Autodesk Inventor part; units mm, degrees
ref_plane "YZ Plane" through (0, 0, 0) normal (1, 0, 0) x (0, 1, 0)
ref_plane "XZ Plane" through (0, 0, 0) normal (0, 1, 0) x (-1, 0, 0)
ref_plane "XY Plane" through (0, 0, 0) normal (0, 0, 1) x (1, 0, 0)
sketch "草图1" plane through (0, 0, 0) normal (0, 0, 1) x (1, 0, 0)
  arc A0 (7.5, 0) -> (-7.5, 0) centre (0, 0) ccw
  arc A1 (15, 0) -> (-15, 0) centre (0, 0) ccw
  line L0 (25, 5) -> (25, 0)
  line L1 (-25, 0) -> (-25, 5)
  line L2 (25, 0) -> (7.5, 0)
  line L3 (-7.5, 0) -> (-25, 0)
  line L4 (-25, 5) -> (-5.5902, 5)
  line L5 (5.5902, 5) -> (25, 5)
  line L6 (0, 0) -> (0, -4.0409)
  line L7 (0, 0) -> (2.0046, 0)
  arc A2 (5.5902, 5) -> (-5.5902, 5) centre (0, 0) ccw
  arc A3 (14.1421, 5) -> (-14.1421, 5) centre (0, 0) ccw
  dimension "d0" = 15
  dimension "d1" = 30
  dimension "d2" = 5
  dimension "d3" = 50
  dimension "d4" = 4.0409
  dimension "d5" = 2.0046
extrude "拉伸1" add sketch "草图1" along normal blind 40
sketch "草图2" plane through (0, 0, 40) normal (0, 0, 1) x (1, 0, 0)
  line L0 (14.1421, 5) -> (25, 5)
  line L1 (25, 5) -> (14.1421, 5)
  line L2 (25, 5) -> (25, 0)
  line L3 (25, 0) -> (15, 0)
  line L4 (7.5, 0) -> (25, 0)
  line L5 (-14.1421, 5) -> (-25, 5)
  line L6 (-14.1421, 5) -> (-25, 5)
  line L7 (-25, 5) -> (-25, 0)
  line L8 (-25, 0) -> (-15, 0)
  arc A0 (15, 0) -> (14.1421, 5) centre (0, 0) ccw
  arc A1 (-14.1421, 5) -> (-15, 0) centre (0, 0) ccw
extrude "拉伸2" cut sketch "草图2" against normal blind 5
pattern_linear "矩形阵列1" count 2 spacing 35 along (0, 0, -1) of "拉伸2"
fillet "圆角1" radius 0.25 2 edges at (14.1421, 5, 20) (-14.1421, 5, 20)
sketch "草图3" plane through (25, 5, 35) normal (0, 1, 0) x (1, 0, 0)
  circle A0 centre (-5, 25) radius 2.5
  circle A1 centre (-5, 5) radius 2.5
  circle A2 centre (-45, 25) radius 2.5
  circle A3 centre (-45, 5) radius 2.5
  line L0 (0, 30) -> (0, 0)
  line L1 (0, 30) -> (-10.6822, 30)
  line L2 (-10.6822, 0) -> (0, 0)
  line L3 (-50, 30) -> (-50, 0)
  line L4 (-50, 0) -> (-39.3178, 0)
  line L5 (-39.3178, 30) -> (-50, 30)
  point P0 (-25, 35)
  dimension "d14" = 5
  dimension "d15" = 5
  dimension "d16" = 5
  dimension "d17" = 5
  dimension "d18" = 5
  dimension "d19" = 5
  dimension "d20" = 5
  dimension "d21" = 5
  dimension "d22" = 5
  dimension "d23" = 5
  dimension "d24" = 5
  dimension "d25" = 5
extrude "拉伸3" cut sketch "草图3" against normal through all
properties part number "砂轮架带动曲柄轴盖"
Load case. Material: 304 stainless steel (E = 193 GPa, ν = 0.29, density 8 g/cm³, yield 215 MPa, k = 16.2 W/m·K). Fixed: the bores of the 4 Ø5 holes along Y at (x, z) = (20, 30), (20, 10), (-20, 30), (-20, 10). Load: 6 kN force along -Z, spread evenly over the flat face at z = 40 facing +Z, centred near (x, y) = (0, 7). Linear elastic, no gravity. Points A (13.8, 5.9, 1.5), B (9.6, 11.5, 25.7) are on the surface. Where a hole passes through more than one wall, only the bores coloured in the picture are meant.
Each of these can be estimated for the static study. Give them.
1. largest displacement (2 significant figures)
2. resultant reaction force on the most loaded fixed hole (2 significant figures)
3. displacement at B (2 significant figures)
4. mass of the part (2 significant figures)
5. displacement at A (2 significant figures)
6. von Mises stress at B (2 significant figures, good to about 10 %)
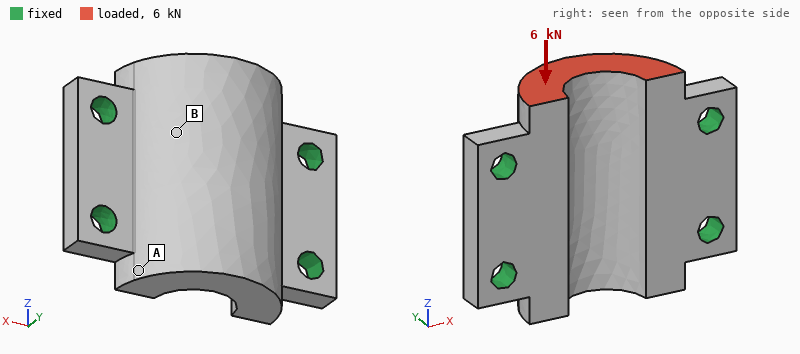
12 µm
2.1 kN
5.9 µm
110 g
4.8 µm
28 MPa
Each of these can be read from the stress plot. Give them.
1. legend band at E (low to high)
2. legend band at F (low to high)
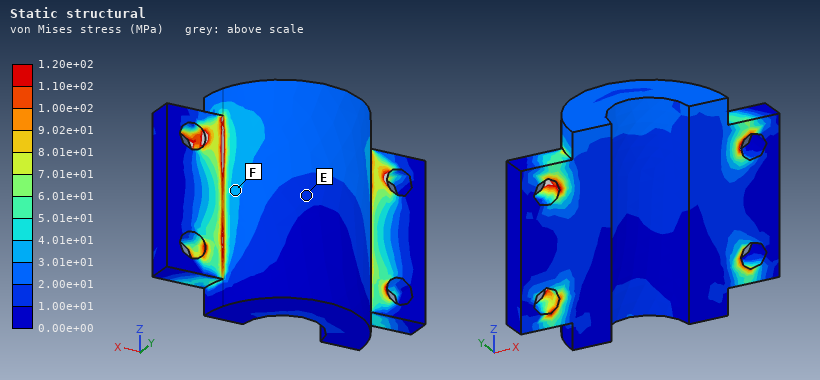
1.00e+01 to 2.00e+01 MPa
3.01e+01 to 4.01e+01 MPa
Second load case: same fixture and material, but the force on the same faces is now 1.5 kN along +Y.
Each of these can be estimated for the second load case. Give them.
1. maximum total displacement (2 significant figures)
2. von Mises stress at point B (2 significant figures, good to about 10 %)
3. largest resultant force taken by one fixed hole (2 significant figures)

10.0 µm
18 MPa
1.3 kN
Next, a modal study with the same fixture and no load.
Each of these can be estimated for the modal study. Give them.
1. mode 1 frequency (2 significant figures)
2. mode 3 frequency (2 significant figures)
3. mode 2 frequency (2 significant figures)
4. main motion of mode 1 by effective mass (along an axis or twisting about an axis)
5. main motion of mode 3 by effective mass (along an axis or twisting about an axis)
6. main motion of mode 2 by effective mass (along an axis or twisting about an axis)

14 kHz
29 kHz
18 kHz
along Z
along Z
along Y
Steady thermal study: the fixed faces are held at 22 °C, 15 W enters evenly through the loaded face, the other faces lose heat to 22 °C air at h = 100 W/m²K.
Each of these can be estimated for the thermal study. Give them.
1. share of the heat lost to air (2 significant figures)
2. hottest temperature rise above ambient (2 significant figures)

42 %
58 K
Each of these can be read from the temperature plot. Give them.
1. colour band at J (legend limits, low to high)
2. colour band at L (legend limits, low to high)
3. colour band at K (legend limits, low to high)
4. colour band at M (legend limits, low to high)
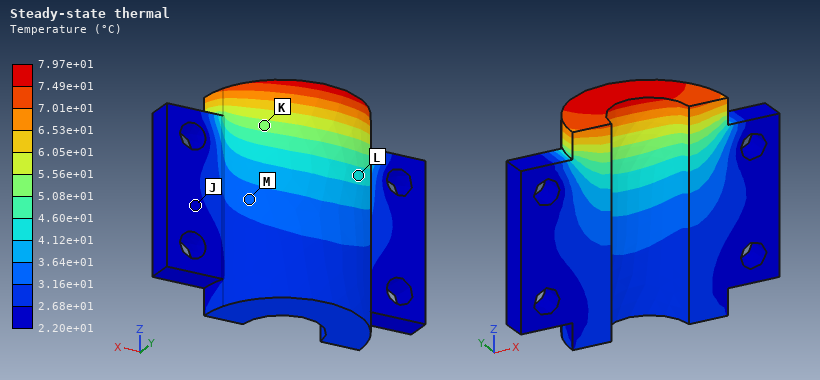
2.20e+01 to 2.68e+01 °C
4.12e+01 to 4.60e+01 °C
5.08e+01 to 5.56e+01 °C
3.16e+01 to 3.64e+01 °C
